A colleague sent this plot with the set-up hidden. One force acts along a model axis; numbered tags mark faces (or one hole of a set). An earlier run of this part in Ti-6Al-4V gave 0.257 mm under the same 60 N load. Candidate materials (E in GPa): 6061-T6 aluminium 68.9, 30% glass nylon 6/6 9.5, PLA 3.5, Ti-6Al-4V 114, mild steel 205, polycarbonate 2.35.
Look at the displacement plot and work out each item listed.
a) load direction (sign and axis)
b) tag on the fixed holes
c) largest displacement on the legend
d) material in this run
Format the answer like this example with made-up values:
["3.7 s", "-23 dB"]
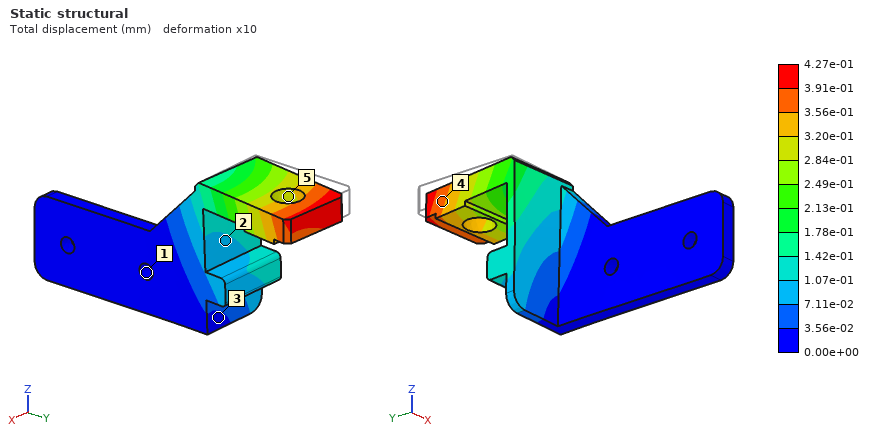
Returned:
["+X", "1", "4.27e-01 mm", "6061-T6 aluminium"]
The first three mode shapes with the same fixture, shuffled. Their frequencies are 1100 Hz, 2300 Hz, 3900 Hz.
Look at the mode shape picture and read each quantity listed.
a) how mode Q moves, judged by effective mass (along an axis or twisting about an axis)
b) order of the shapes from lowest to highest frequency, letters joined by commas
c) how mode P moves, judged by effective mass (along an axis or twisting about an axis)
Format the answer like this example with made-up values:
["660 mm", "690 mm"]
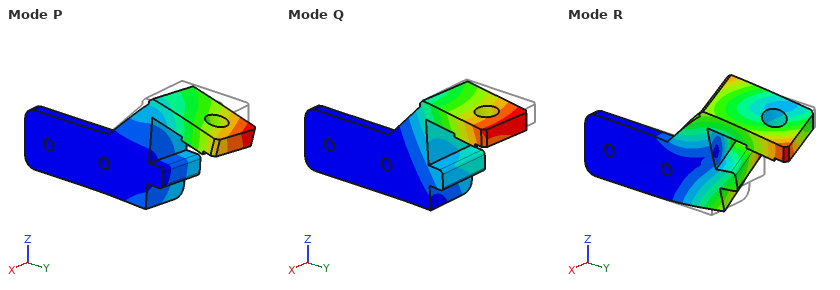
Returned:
["along X", "Q, P, R", "along Z"]
